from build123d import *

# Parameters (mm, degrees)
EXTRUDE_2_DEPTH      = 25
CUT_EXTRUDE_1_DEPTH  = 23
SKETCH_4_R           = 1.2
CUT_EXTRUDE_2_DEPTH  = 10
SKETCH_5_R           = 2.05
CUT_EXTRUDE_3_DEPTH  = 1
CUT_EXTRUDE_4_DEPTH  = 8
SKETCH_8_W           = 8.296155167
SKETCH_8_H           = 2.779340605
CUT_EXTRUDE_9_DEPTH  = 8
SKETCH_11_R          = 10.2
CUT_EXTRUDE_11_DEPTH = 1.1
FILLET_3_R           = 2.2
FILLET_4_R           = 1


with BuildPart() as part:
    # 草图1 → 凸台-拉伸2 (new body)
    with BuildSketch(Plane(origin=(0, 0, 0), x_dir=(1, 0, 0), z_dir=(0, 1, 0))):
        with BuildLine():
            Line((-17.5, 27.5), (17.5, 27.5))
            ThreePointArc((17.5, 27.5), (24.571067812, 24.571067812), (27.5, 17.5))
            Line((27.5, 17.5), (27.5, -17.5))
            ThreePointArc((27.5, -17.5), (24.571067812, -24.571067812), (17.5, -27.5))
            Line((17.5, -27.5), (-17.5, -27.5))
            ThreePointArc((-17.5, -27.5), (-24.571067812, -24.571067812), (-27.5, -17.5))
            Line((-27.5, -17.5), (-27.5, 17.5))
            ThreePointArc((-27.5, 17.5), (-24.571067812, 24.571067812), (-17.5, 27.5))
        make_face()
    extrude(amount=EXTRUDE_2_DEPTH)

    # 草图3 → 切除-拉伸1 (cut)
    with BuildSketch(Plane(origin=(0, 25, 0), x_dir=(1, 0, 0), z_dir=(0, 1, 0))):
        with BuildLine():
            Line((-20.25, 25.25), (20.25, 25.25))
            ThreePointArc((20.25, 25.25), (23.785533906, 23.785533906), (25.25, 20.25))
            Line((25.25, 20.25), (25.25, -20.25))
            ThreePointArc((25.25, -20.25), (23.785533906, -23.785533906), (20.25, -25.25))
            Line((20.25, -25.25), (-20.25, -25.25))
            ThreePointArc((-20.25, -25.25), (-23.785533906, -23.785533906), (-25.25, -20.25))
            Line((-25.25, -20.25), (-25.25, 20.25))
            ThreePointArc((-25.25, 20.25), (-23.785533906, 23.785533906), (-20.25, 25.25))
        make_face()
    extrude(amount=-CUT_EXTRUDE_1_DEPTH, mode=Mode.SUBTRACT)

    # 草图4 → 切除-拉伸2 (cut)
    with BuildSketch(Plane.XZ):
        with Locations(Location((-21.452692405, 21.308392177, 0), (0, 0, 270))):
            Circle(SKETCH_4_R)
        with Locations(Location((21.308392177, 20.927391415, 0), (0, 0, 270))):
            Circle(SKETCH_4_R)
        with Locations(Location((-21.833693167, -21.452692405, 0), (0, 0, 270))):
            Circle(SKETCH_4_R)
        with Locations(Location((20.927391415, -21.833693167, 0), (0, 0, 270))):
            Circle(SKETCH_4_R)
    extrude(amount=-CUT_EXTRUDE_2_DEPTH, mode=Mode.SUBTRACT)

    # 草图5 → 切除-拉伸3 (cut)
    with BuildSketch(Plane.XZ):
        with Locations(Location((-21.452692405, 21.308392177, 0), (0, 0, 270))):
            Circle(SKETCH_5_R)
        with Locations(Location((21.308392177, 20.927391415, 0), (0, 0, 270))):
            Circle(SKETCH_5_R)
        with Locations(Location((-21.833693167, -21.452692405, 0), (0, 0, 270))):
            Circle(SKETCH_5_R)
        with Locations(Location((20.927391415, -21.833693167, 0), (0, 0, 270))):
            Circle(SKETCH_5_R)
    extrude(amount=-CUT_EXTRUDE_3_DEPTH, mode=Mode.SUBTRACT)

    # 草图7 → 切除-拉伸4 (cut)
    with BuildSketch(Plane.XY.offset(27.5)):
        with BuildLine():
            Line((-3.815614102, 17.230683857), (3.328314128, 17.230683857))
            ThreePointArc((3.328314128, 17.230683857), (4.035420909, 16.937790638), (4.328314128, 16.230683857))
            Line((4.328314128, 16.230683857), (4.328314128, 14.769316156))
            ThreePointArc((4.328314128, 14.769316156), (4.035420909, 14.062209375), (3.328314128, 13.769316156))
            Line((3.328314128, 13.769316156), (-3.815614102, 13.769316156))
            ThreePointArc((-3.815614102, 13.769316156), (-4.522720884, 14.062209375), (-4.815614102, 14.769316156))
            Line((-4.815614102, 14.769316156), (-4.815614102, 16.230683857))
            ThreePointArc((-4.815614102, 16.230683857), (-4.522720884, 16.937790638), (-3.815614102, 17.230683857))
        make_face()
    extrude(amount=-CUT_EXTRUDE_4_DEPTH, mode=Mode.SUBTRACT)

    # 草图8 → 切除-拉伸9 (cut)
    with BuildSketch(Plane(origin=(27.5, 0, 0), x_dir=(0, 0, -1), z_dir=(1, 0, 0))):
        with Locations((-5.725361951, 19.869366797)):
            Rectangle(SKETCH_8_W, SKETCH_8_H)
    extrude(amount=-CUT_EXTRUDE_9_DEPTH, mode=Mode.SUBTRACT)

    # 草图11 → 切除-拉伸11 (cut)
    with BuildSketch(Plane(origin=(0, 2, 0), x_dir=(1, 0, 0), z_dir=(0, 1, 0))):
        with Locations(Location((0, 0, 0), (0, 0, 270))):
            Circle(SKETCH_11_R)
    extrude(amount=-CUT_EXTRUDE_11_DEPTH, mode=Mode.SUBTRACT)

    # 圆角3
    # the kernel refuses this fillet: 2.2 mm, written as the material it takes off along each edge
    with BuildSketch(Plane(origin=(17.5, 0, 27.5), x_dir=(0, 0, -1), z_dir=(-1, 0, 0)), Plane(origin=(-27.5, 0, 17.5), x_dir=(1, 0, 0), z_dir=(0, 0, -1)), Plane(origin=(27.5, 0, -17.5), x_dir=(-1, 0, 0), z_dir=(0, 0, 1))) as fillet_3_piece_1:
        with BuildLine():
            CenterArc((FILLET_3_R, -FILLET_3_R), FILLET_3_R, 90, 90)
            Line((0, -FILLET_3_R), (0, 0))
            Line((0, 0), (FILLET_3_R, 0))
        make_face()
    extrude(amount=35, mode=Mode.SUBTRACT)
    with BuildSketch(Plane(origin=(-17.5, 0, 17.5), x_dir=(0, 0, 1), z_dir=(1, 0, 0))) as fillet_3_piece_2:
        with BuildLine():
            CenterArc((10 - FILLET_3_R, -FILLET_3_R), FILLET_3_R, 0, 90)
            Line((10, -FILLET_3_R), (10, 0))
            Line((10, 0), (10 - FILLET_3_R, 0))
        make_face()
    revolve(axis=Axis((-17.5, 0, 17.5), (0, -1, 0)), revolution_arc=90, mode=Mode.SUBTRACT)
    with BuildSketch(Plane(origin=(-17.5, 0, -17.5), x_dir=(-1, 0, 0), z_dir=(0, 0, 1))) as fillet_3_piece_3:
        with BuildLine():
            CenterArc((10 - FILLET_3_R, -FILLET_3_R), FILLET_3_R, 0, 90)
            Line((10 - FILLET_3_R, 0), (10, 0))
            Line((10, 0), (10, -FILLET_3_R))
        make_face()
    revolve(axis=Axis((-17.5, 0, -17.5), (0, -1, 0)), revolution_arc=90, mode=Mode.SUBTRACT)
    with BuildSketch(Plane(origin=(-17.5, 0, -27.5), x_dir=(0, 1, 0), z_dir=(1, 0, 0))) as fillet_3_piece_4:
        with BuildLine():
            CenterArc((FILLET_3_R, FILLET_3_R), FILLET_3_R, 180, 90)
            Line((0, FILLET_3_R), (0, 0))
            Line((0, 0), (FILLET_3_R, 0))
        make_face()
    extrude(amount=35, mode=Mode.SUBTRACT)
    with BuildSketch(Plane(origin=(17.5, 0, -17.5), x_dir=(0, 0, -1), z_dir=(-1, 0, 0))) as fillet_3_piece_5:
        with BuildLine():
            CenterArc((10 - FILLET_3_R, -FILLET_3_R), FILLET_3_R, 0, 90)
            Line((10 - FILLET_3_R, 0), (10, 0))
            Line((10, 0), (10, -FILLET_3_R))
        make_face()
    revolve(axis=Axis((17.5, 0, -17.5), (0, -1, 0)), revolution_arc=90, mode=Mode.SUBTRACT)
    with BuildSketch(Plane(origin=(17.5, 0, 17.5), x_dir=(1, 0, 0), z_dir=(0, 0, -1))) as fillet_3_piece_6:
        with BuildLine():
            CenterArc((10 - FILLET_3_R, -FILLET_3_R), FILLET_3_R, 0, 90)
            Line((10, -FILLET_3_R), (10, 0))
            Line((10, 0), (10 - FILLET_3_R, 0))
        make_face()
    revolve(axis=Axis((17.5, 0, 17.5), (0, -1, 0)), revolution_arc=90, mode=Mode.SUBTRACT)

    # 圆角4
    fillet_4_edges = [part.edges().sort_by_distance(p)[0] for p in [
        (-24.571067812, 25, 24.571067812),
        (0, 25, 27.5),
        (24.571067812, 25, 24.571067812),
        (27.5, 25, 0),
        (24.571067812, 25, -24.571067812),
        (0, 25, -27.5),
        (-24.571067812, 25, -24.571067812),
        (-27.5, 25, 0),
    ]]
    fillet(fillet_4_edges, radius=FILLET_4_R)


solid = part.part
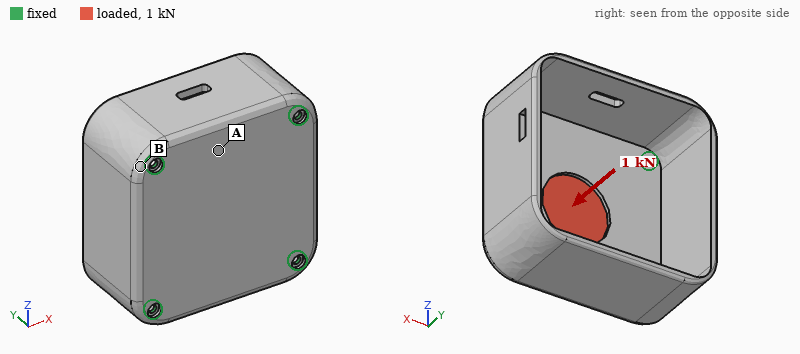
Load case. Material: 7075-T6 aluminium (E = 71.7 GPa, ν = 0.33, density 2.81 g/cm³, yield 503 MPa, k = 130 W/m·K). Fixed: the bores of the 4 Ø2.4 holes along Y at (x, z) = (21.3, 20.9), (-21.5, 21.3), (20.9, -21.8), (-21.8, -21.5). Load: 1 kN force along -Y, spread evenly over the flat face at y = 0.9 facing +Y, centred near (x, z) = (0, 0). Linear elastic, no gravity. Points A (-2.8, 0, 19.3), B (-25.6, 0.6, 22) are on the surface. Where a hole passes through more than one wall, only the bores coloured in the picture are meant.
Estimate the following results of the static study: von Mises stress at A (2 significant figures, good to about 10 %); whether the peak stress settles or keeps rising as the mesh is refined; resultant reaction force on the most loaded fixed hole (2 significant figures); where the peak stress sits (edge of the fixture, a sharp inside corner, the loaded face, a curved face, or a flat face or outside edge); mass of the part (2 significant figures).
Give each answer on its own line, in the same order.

67 MPa
keeps rising
450 N
edge of the fixture
41 g
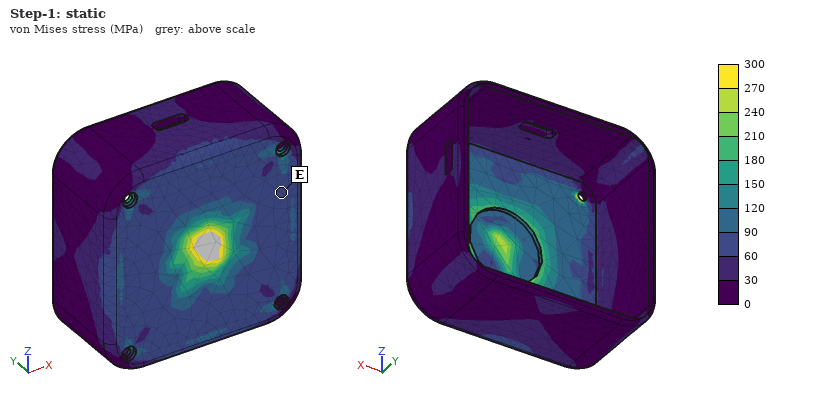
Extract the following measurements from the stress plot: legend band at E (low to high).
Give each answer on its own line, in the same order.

60 to 90 MPa
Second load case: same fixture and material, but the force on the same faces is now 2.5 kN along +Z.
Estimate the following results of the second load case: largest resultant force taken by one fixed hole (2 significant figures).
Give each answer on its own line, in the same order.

660 N
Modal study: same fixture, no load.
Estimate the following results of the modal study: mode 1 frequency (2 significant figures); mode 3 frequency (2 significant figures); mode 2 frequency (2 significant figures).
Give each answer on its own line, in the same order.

3500 Hz
4100 Hz
4100 Hz
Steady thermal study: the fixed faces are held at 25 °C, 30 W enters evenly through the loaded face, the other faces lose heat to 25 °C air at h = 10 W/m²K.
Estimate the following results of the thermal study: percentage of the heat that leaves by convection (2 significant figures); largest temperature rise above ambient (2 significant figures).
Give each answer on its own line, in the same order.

7.1 %
52 K
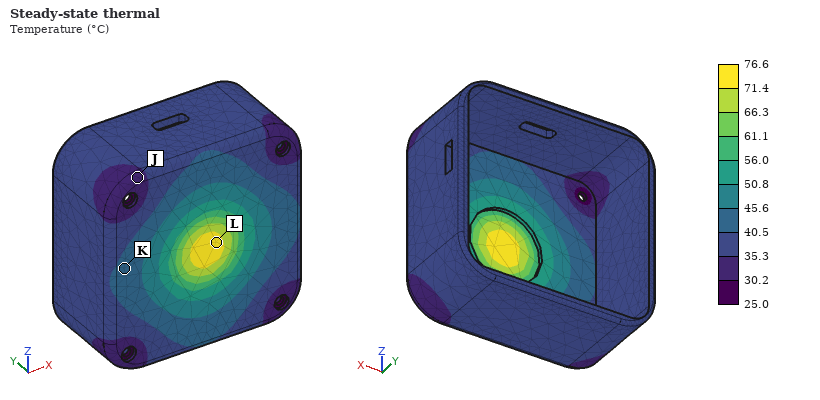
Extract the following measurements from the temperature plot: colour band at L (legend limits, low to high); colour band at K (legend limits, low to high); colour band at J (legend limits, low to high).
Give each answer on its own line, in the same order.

71.4 to 76.6 °C
40.5 to 45.6 °C
30.2 to 35.3 °C
